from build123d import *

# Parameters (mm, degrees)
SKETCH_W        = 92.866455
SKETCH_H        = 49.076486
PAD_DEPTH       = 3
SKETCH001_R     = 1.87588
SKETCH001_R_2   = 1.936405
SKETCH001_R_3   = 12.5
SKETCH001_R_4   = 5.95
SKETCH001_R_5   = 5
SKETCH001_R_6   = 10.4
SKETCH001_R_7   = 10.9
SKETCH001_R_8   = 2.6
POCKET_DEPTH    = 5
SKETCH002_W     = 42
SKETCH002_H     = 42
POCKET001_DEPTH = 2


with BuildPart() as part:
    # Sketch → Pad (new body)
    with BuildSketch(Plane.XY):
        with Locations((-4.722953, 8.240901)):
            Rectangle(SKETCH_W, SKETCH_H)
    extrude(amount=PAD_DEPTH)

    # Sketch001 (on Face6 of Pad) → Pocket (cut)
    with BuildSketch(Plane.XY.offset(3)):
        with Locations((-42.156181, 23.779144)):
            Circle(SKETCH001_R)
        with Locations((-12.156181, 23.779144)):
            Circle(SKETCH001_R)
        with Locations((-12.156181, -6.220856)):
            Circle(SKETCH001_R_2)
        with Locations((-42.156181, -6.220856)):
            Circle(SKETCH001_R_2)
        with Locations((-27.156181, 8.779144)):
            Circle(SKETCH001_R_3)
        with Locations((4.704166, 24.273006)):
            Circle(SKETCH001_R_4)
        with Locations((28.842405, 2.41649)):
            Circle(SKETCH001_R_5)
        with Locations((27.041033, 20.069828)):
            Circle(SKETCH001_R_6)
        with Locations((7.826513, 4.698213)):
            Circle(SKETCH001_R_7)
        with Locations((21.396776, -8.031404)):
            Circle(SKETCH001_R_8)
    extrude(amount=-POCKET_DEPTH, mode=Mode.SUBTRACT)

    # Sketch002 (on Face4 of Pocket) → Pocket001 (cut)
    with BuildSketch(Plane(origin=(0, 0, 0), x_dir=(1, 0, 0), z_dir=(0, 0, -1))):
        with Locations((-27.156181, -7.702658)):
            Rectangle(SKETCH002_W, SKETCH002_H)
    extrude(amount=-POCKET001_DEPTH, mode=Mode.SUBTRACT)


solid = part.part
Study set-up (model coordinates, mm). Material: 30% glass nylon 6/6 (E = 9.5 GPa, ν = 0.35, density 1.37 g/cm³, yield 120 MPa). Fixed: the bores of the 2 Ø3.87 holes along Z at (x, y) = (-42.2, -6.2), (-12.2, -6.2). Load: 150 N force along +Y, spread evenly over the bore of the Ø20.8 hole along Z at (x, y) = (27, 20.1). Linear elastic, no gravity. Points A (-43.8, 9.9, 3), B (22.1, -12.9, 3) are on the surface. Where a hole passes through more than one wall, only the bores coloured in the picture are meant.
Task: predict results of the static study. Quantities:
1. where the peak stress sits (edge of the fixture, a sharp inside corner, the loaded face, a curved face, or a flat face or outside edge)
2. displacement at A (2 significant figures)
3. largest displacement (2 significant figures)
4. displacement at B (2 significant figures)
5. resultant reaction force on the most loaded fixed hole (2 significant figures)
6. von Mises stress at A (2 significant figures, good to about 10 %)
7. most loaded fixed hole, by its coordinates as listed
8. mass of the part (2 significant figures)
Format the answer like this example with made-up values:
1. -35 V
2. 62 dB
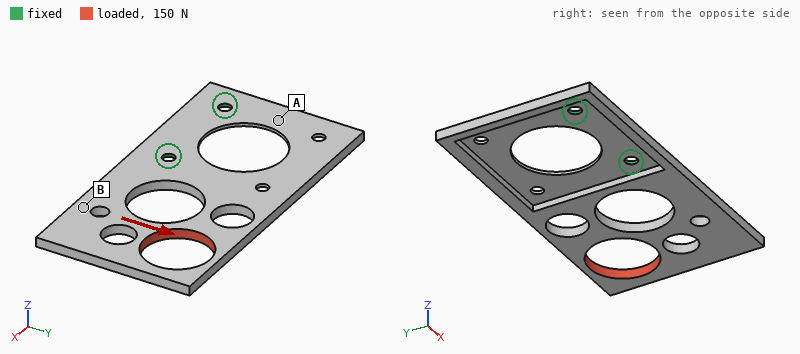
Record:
1. edge of the fixture
2. 0.23 mm
3. 0.76 mm
4. 0.38 mm
5. 310 N
6. 15 MPa
7. (-12.2, -6.2)
8. 9.4 g
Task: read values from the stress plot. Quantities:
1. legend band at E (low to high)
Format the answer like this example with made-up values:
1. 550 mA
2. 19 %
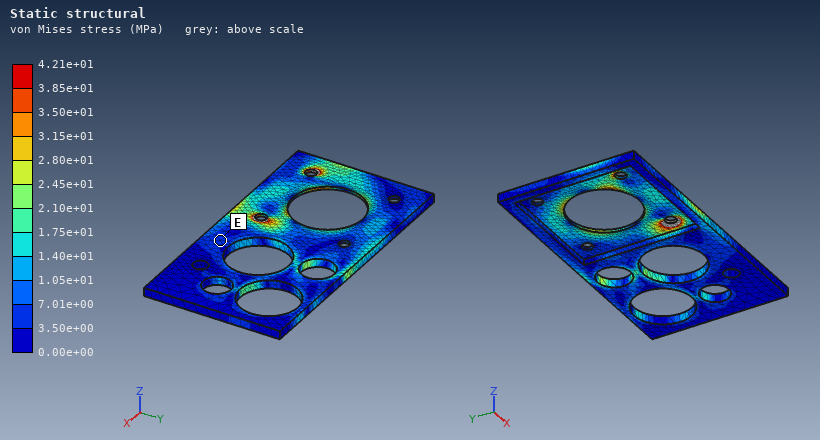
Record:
1. 3.50e+00 to 7.01e+00 MPa
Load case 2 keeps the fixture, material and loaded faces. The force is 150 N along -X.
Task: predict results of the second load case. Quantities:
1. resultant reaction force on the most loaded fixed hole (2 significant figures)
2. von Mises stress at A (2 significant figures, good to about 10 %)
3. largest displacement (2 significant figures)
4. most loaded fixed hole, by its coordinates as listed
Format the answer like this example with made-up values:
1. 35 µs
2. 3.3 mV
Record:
1. 140 N
2. 11 MPa
3. 1.00 mm
4. (-12.2, -6.2)
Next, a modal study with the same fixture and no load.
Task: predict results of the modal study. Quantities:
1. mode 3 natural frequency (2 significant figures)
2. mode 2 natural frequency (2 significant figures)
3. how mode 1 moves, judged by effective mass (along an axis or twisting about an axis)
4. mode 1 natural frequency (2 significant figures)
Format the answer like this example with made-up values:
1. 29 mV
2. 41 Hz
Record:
1. 630 Hz
2. 310 Hz
3. along Z
4. 190 Hz
